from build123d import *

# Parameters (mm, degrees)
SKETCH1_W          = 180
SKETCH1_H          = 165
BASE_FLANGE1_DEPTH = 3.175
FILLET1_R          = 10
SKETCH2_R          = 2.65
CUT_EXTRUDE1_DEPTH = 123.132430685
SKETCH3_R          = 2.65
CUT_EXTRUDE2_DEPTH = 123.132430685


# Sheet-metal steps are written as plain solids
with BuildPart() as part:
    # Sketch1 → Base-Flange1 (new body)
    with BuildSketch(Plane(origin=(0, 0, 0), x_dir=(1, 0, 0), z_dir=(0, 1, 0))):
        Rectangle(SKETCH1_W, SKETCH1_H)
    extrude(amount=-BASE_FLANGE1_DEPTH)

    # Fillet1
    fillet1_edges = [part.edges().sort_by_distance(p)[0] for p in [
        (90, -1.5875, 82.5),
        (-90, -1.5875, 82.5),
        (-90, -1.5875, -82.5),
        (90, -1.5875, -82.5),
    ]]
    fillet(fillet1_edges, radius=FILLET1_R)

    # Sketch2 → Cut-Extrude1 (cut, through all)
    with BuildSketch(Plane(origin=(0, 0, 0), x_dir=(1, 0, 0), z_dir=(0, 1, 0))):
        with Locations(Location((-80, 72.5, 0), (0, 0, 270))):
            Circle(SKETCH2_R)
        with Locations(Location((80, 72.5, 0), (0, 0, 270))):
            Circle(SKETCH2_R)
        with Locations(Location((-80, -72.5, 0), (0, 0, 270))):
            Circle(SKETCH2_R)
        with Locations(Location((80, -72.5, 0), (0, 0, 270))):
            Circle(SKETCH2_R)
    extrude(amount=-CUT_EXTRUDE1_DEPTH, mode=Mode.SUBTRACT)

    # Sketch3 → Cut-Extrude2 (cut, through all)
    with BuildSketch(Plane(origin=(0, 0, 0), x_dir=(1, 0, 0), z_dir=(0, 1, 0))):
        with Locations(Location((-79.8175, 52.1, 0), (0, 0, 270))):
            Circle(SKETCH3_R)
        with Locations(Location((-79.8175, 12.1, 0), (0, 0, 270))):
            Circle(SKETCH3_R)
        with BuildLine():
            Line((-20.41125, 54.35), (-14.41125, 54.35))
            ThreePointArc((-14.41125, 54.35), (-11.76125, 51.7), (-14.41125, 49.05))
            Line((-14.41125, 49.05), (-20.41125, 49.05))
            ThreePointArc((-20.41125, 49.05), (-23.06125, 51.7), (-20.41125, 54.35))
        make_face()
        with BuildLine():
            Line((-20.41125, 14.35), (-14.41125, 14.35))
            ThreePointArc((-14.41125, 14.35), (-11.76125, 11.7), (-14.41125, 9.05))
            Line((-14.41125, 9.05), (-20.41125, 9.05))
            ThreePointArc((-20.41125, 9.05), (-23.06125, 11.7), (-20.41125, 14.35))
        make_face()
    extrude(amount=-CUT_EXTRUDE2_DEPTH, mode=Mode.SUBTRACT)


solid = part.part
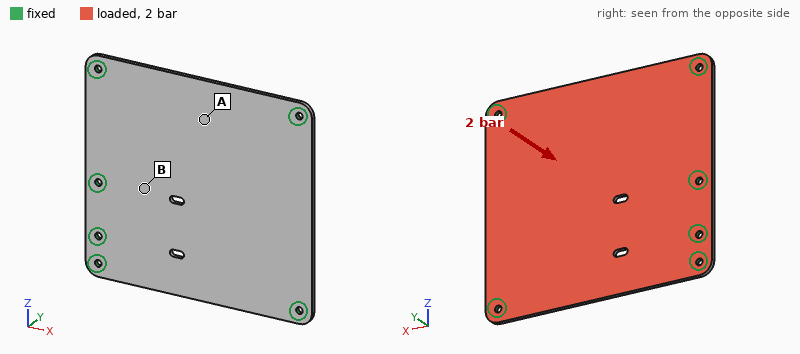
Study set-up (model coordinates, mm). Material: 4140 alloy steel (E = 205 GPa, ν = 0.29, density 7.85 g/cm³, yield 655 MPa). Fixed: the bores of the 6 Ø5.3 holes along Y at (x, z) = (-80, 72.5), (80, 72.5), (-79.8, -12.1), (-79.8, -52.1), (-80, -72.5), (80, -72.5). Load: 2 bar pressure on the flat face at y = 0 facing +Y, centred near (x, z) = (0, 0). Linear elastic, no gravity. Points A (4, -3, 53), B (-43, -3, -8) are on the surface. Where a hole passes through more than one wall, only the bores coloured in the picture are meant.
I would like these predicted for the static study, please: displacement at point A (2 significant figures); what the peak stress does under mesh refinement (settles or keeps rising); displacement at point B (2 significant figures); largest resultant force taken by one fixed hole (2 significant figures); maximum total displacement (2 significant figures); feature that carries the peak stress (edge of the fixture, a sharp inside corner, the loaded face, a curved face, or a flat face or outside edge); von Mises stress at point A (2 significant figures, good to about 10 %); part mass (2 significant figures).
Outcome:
0.96 mm
keeps rising
0.50 mm
1.4 kN
1.1 mm
edge of the fixture
150 MPa
730 g
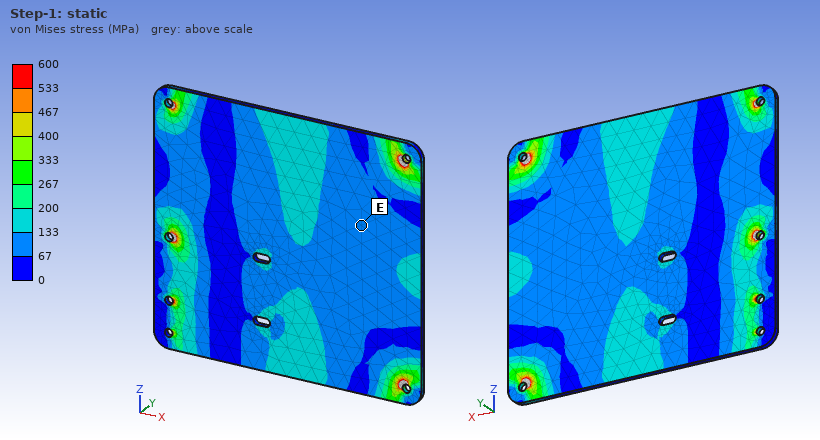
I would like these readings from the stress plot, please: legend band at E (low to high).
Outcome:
67 to 133 MPa
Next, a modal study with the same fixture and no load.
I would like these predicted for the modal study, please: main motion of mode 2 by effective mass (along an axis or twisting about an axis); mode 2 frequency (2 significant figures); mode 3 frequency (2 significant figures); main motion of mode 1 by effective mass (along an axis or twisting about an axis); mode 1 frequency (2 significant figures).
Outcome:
twisting about X
750 Hz
870 Hz
along Y
510 Hz
